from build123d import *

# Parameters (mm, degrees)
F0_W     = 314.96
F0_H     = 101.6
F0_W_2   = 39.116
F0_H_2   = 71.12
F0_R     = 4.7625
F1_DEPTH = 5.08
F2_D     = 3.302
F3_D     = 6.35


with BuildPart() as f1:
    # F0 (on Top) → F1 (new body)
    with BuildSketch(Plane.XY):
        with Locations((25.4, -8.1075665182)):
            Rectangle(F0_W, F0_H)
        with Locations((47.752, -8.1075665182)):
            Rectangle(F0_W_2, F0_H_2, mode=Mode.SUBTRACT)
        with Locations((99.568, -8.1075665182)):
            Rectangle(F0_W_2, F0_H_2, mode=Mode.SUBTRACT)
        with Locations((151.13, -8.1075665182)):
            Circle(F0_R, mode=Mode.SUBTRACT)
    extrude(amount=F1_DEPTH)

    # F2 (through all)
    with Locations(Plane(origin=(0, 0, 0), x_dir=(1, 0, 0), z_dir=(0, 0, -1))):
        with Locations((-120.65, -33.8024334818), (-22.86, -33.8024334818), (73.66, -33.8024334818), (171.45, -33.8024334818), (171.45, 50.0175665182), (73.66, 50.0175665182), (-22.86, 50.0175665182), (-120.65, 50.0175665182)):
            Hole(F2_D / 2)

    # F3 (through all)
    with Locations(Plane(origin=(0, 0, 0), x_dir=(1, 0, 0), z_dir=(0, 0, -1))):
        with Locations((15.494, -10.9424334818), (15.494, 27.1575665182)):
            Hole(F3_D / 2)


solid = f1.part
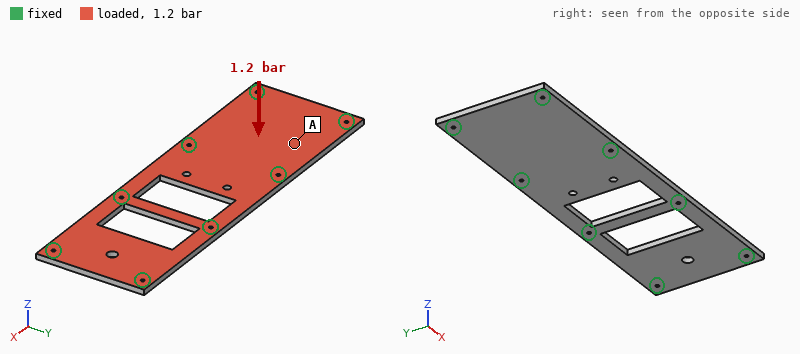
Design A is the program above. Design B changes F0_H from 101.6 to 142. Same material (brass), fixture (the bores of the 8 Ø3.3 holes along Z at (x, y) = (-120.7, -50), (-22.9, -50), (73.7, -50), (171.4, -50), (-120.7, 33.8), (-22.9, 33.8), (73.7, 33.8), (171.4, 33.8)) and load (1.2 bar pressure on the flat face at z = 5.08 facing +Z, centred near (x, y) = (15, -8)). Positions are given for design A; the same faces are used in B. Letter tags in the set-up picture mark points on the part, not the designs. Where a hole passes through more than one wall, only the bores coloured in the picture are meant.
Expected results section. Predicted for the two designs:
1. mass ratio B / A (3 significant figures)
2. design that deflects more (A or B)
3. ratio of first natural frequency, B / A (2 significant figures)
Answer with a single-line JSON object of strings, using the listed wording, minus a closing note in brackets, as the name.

{"mass ratio B / A": "1.49", "design that deflects more": "A", "ratio of first natural frequency, B / A": "1.0"}
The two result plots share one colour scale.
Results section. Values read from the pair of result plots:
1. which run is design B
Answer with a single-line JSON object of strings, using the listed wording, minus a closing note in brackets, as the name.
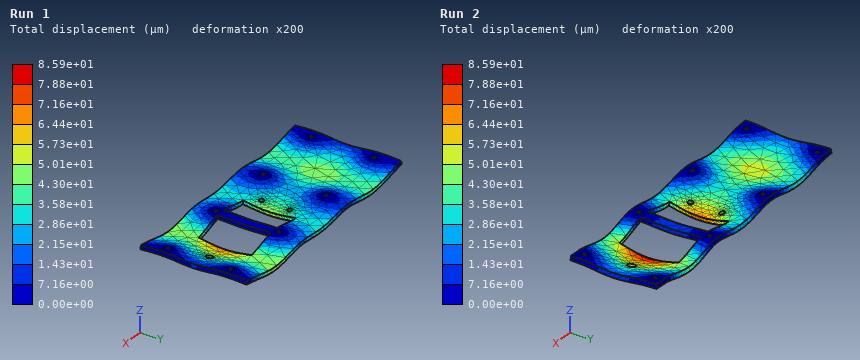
{"which run is design B": "Run 1"}
